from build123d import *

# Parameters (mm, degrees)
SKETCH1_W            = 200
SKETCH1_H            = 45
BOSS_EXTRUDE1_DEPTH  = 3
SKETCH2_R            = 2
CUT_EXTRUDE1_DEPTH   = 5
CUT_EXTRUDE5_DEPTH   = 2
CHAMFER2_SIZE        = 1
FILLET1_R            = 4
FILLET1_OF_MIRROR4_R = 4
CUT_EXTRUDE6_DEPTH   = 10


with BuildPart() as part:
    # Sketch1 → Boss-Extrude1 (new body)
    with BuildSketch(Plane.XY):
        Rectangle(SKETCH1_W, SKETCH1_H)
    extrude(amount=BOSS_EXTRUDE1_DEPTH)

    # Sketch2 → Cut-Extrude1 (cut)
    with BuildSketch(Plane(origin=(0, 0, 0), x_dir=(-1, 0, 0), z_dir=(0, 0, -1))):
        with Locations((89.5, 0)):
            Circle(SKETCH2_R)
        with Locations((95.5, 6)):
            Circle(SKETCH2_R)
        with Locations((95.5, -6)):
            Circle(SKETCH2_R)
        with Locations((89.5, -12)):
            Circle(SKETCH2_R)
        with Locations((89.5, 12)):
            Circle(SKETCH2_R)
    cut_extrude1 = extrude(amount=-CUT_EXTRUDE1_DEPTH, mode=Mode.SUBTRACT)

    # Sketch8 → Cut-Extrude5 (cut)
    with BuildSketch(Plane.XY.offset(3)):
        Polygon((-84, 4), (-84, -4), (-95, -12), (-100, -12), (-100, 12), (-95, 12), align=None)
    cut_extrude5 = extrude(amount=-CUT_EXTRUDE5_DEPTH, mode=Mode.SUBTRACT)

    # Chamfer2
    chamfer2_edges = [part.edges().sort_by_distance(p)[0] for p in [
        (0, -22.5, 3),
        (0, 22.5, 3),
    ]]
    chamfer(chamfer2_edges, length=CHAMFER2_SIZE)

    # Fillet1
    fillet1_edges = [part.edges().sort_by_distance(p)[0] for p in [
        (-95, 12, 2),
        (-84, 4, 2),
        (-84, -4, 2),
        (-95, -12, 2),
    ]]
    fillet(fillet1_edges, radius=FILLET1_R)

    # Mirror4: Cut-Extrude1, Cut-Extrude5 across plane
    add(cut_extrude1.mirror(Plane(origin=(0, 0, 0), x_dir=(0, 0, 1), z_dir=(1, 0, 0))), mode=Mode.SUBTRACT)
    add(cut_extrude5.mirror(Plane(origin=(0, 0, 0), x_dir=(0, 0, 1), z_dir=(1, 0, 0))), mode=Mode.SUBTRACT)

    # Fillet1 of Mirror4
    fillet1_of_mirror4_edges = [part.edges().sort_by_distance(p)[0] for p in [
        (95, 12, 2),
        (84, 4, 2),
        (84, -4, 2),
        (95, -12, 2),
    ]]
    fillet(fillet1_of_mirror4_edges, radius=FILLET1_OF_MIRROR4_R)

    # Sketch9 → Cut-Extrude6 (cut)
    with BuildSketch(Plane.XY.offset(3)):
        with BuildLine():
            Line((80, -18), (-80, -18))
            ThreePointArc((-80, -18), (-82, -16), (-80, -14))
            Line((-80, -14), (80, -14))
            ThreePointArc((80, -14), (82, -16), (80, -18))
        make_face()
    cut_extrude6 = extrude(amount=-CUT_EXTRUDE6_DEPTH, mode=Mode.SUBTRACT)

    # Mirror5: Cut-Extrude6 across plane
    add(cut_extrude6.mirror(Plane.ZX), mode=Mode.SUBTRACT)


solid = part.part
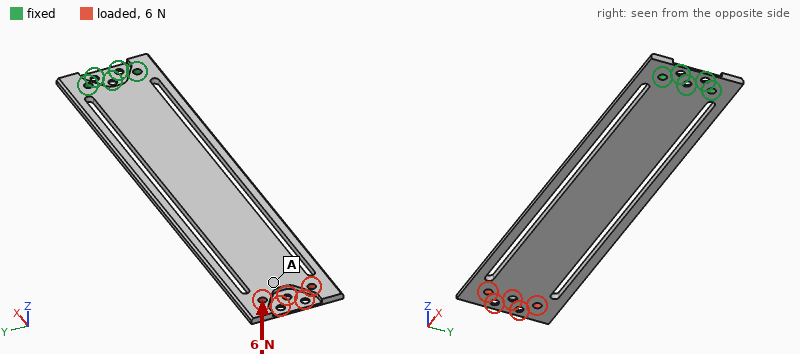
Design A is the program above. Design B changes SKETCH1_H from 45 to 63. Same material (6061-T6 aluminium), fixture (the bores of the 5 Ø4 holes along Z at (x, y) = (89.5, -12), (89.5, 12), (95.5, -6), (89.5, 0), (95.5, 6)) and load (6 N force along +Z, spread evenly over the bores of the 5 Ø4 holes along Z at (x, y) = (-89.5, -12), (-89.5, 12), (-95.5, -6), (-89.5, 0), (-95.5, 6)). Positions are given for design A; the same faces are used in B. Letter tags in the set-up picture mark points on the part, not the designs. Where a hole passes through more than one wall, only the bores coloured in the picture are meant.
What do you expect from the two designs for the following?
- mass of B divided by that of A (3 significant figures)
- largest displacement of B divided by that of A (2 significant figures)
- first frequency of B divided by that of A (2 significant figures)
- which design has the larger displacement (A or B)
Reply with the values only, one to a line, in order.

1.50
0.69
0.98
A
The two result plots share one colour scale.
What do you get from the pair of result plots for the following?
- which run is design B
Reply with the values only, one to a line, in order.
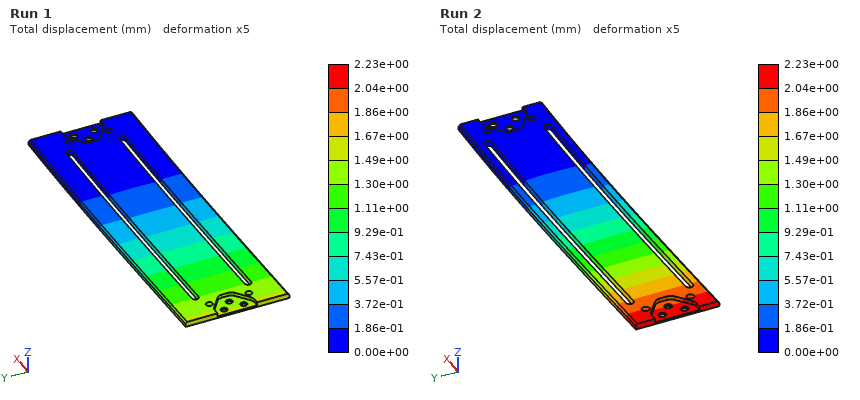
Run 1
